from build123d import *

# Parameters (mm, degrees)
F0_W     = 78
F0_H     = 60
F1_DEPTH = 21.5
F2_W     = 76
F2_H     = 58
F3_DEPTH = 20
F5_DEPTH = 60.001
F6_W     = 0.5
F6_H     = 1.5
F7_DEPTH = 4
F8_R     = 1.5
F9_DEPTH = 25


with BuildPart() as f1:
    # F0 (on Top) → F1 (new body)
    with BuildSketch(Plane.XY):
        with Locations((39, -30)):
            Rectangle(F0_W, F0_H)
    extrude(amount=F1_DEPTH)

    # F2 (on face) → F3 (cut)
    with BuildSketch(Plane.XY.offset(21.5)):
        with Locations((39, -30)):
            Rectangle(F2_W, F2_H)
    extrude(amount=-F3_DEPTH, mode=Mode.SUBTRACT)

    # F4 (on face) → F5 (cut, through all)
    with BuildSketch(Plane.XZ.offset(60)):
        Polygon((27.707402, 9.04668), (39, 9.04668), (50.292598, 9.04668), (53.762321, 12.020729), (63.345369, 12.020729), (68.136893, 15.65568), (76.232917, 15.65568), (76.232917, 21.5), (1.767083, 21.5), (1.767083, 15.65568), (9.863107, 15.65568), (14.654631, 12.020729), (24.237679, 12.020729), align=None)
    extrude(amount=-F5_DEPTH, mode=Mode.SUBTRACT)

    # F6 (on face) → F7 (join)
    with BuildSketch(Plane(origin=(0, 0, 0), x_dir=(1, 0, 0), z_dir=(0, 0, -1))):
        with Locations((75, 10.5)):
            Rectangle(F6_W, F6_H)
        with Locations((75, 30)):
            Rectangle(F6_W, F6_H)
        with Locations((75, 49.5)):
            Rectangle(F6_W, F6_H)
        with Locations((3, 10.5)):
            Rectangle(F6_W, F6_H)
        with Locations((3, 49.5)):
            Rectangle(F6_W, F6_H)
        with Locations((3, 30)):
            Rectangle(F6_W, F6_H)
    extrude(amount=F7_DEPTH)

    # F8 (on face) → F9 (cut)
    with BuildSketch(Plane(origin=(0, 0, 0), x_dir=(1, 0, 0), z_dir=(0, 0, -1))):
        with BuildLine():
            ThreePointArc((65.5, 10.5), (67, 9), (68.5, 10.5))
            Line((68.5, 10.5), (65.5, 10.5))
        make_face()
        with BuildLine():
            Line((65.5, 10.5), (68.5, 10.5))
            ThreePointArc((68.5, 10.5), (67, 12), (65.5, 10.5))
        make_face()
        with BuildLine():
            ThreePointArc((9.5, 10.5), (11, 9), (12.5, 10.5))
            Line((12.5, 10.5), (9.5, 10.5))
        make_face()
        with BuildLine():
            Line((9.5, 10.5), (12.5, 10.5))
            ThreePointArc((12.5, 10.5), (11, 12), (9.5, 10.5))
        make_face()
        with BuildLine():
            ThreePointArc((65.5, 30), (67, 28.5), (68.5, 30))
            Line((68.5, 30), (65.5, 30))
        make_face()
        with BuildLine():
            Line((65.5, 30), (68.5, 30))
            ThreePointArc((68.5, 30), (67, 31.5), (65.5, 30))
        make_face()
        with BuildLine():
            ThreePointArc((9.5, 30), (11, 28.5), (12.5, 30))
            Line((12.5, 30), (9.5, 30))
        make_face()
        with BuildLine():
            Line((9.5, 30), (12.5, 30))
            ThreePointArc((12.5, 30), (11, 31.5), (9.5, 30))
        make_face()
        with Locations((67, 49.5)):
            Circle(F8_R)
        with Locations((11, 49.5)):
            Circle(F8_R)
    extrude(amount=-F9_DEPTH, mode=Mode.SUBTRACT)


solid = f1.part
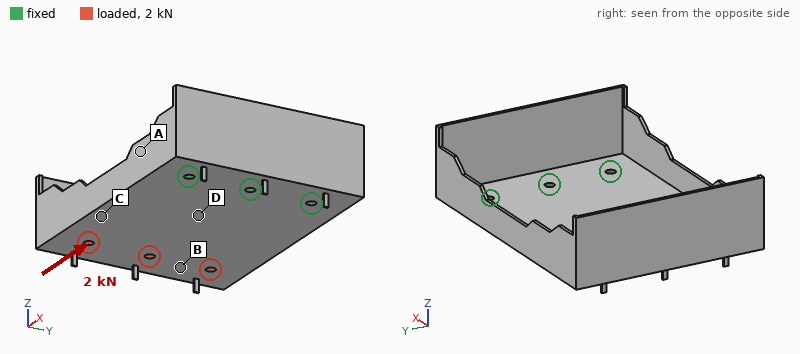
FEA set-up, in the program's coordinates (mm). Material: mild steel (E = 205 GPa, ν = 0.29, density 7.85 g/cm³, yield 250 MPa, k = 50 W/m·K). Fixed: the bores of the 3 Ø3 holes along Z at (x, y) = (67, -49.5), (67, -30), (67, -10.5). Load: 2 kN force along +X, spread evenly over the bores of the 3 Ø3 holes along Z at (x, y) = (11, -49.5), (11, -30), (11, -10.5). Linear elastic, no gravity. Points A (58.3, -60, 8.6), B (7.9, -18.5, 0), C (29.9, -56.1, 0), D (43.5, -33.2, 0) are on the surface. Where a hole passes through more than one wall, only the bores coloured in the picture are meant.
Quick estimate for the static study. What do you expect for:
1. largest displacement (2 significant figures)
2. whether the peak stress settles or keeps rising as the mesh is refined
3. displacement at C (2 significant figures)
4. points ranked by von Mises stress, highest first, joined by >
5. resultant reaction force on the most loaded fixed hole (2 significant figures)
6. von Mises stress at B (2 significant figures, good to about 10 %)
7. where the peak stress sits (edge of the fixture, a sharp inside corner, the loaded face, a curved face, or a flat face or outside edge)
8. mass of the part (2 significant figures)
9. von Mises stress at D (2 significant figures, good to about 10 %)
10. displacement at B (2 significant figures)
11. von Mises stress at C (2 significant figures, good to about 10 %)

22 µm
keeps rising
7.4 µm
D > C > B > A
710 N
12 MPa
edge of the fixture
86 g
26 MPa
18 µm
21 MPa
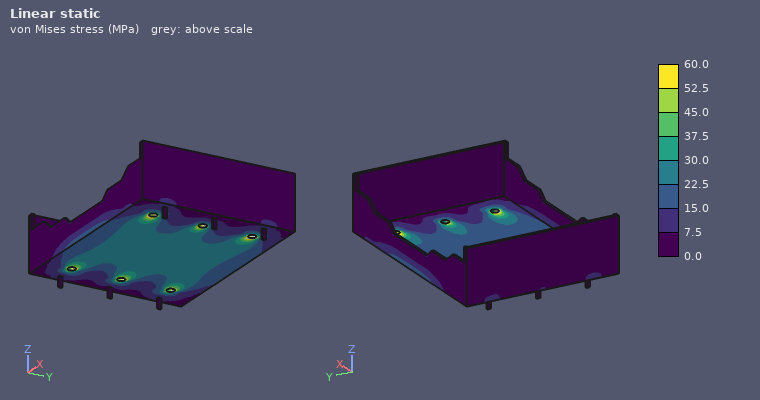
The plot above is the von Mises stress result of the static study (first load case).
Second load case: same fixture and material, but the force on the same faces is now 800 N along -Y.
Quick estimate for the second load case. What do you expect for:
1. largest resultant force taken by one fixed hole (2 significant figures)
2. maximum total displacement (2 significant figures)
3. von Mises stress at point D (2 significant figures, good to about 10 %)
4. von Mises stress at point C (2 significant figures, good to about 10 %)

1.1 kN
36 µm
23 MPa
15 MPa
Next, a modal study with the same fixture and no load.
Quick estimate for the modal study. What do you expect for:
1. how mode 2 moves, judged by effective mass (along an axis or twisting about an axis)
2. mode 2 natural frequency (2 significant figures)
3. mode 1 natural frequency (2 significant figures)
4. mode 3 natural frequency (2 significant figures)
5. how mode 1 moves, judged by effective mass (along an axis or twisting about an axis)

twisting about X
600 Hz
390 Hz
2100 Hz
along Z
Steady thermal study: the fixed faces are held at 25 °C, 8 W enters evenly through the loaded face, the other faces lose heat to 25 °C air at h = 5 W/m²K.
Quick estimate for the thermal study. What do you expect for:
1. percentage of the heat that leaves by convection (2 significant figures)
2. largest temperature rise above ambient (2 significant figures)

36 %
72 K
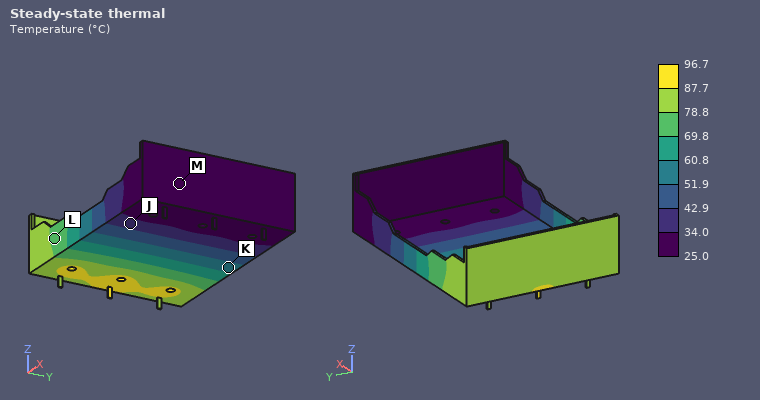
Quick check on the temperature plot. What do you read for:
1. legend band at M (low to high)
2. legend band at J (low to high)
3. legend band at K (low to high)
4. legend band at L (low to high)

25.0 to 34.0 °C
34.0 to 42.9 °C
51.9 to 60.8 °C
69.8 to 78.8 °C
